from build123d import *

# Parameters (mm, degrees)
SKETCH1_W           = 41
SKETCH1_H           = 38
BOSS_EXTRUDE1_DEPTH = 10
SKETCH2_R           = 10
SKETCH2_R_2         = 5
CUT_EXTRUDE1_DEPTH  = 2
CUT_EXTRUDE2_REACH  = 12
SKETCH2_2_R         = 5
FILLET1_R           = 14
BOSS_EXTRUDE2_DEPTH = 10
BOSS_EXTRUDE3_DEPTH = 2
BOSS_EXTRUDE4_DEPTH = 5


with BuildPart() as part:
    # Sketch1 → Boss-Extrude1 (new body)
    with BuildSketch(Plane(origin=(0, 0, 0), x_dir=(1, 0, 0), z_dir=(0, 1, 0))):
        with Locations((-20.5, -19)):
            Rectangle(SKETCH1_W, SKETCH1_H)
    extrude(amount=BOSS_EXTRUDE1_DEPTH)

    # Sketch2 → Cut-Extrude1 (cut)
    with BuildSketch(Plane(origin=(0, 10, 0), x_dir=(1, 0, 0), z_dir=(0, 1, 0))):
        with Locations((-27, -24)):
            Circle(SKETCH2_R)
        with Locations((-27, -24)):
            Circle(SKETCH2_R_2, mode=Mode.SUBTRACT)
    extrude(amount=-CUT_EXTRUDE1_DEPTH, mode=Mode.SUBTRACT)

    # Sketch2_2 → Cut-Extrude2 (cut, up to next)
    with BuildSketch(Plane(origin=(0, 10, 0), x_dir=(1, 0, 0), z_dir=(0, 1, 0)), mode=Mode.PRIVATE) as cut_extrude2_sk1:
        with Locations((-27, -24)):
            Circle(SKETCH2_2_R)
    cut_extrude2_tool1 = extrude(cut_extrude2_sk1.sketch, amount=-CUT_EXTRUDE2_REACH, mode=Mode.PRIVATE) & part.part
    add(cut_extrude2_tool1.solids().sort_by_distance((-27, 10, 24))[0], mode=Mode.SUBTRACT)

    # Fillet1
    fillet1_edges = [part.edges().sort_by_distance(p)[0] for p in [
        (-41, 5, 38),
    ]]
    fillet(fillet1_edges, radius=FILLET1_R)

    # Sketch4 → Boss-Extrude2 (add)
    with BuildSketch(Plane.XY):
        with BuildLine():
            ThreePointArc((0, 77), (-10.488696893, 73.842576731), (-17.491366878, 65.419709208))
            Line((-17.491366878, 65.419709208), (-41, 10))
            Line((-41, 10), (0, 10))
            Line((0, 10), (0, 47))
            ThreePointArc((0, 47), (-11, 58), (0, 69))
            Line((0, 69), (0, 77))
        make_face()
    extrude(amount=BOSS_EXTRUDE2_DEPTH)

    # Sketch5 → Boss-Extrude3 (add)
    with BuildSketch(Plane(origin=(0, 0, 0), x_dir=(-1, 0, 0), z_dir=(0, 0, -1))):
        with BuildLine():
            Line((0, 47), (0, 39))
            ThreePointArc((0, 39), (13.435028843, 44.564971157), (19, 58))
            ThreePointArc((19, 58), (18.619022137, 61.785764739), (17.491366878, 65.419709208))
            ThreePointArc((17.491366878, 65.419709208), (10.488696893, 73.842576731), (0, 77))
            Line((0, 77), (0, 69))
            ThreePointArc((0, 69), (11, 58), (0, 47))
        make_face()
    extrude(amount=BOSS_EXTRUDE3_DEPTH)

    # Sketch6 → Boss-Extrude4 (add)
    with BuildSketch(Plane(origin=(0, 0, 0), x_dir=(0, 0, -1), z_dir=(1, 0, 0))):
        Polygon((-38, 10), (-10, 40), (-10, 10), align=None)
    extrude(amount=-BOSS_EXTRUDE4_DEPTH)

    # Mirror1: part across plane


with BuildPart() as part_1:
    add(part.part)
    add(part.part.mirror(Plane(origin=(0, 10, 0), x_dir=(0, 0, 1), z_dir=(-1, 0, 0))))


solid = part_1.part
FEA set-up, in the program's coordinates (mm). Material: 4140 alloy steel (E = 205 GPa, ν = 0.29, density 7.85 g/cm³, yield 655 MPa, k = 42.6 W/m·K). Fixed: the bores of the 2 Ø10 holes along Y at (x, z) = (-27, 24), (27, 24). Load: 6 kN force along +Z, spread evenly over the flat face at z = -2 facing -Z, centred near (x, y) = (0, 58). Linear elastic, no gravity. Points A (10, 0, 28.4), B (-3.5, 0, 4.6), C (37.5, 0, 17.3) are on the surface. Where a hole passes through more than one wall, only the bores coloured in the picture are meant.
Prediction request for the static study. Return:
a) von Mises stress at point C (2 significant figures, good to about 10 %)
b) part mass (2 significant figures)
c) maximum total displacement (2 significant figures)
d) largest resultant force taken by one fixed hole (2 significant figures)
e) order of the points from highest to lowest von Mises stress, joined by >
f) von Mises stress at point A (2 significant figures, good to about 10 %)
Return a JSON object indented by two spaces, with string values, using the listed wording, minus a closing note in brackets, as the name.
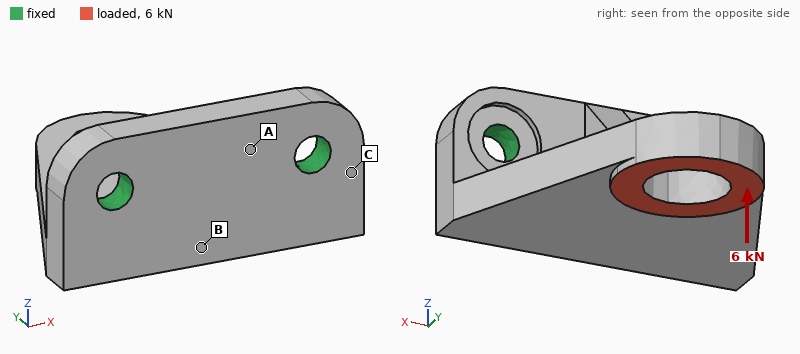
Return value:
{
  "von Mises stress at point C": "150 MPa",
  "part mass": "510 g",
  "maximum total displacement": "0.42 mm",
  "largest resultant force taken by one fixed hole": "3.6 kN",
  "order of the points from highest to lowest von Mises stress, joined by >": "C > A > B",
  "von Mises stress at point A": "97 MPa"
}
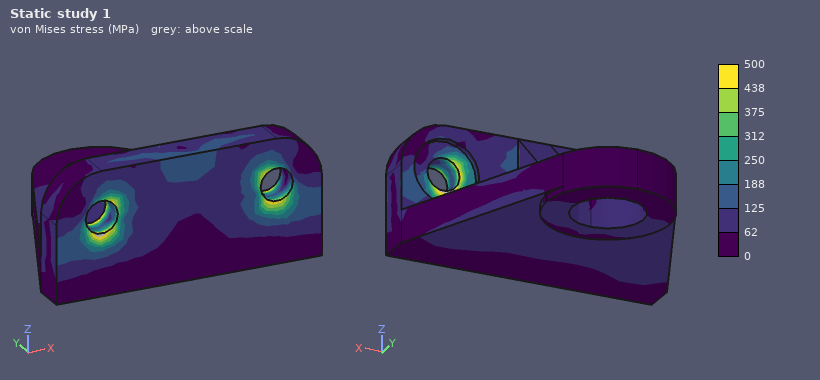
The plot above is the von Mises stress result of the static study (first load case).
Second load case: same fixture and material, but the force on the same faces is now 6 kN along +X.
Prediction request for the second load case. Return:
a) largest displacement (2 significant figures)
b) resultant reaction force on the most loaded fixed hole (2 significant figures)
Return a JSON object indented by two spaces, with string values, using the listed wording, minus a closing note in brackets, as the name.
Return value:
{
  "largest displacement": "58 µm",
  "resultant reaction force on the most loaded fixed hole": "7.0 kN"
}
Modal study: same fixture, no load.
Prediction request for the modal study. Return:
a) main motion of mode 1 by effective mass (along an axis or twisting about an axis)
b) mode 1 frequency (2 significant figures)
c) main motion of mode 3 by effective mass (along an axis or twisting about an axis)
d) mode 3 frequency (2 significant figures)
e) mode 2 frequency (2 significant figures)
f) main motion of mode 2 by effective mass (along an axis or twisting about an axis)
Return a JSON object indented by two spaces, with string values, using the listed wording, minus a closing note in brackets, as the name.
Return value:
{
  "main motion of mode 1 by effective mass": "along Z",
  "mode 1 frequency": "2200 Hz",
  "main motion of mode 3 by effective mass": "along Y",
  "mode 3 frequency": "6500 Hz",
  "mode 2 frequency": "5000 Hz",
  "main motion of mode 2 by effective mass": "along X"
}
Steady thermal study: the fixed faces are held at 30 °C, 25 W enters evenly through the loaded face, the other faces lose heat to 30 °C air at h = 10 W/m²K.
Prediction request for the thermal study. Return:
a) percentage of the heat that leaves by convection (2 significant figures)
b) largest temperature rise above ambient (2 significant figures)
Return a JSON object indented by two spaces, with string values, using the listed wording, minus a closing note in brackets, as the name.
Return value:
{
  "percentage of the heat that leaves by convection": "14 %",
  "largest temperature rise above ambient": "74 K"
}
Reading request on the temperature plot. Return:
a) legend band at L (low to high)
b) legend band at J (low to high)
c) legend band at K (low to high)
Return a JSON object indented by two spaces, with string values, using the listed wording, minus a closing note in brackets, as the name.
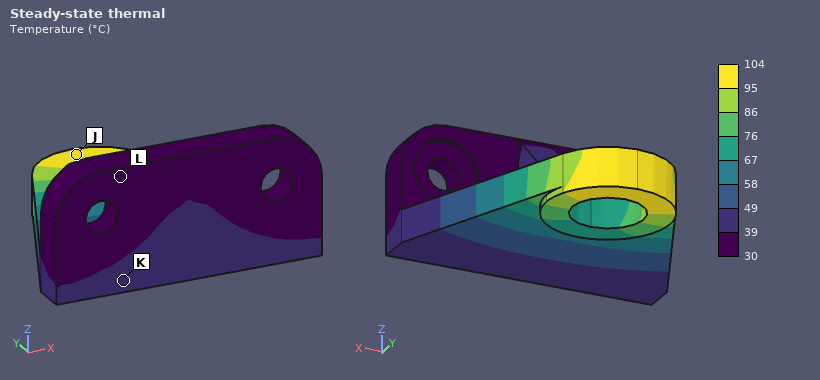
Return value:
{
  "legend band at L": "30 to 39 °C",
  "legend band at J": "95 to 104 °C",
  "legend band at K": "39 to 49 °C"
}
